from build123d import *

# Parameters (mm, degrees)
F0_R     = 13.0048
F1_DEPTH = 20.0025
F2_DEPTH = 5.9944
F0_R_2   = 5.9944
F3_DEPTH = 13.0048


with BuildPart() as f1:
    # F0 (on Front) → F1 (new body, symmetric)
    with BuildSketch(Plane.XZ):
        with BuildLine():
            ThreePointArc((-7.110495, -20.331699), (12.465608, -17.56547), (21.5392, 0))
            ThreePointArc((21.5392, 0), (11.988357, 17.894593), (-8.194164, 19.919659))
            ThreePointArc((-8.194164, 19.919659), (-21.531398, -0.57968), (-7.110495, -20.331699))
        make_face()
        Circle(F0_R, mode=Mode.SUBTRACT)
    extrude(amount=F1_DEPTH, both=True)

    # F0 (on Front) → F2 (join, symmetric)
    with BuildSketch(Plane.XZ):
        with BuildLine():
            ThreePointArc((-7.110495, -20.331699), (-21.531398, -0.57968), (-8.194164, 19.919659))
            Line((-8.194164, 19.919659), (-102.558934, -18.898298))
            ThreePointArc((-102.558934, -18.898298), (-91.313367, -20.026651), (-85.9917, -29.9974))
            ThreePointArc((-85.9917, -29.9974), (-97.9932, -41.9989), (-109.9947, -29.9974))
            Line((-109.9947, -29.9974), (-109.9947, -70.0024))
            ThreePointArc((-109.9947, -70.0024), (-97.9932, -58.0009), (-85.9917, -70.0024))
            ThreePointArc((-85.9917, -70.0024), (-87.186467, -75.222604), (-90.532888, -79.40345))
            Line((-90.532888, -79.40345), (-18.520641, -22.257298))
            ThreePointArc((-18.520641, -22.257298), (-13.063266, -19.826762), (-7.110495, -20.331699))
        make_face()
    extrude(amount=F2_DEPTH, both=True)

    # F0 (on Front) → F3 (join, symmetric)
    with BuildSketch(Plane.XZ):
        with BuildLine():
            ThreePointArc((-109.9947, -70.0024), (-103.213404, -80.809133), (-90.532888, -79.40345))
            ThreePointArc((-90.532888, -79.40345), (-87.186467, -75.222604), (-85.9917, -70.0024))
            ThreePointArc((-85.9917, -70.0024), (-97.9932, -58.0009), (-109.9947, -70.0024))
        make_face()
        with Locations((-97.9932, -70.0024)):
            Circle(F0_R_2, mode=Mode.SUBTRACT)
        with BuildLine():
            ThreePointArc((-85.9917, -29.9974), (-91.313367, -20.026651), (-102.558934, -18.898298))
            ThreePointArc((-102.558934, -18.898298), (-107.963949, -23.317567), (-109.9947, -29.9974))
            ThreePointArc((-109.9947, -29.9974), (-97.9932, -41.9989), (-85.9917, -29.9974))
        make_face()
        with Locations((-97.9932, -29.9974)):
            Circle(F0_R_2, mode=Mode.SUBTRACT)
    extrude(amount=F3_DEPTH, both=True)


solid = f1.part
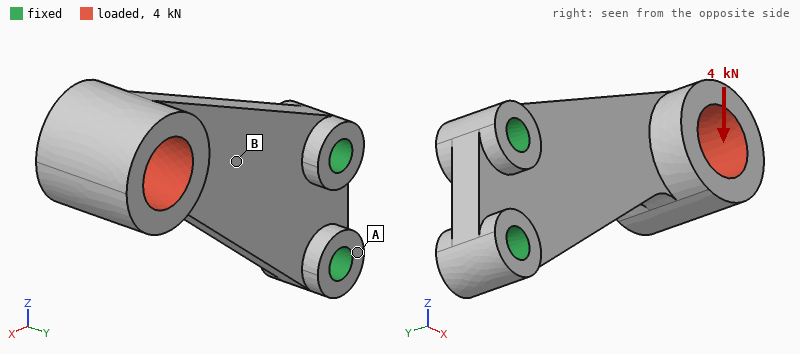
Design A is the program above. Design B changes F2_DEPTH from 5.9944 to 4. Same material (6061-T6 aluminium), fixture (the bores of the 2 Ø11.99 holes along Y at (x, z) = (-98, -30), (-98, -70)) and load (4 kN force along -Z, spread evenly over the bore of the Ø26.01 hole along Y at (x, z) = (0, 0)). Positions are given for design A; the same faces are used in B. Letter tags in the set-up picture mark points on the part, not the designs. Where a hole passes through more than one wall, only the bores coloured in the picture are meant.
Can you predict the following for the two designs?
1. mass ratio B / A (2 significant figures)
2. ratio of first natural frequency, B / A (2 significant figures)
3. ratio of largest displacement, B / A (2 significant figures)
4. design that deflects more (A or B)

0.84
0.57
1.4
B
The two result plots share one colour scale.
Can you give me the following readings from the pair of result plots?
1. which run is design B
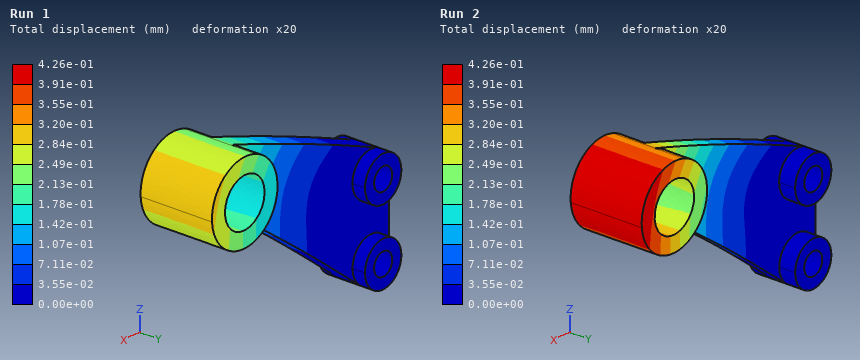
Run 2
